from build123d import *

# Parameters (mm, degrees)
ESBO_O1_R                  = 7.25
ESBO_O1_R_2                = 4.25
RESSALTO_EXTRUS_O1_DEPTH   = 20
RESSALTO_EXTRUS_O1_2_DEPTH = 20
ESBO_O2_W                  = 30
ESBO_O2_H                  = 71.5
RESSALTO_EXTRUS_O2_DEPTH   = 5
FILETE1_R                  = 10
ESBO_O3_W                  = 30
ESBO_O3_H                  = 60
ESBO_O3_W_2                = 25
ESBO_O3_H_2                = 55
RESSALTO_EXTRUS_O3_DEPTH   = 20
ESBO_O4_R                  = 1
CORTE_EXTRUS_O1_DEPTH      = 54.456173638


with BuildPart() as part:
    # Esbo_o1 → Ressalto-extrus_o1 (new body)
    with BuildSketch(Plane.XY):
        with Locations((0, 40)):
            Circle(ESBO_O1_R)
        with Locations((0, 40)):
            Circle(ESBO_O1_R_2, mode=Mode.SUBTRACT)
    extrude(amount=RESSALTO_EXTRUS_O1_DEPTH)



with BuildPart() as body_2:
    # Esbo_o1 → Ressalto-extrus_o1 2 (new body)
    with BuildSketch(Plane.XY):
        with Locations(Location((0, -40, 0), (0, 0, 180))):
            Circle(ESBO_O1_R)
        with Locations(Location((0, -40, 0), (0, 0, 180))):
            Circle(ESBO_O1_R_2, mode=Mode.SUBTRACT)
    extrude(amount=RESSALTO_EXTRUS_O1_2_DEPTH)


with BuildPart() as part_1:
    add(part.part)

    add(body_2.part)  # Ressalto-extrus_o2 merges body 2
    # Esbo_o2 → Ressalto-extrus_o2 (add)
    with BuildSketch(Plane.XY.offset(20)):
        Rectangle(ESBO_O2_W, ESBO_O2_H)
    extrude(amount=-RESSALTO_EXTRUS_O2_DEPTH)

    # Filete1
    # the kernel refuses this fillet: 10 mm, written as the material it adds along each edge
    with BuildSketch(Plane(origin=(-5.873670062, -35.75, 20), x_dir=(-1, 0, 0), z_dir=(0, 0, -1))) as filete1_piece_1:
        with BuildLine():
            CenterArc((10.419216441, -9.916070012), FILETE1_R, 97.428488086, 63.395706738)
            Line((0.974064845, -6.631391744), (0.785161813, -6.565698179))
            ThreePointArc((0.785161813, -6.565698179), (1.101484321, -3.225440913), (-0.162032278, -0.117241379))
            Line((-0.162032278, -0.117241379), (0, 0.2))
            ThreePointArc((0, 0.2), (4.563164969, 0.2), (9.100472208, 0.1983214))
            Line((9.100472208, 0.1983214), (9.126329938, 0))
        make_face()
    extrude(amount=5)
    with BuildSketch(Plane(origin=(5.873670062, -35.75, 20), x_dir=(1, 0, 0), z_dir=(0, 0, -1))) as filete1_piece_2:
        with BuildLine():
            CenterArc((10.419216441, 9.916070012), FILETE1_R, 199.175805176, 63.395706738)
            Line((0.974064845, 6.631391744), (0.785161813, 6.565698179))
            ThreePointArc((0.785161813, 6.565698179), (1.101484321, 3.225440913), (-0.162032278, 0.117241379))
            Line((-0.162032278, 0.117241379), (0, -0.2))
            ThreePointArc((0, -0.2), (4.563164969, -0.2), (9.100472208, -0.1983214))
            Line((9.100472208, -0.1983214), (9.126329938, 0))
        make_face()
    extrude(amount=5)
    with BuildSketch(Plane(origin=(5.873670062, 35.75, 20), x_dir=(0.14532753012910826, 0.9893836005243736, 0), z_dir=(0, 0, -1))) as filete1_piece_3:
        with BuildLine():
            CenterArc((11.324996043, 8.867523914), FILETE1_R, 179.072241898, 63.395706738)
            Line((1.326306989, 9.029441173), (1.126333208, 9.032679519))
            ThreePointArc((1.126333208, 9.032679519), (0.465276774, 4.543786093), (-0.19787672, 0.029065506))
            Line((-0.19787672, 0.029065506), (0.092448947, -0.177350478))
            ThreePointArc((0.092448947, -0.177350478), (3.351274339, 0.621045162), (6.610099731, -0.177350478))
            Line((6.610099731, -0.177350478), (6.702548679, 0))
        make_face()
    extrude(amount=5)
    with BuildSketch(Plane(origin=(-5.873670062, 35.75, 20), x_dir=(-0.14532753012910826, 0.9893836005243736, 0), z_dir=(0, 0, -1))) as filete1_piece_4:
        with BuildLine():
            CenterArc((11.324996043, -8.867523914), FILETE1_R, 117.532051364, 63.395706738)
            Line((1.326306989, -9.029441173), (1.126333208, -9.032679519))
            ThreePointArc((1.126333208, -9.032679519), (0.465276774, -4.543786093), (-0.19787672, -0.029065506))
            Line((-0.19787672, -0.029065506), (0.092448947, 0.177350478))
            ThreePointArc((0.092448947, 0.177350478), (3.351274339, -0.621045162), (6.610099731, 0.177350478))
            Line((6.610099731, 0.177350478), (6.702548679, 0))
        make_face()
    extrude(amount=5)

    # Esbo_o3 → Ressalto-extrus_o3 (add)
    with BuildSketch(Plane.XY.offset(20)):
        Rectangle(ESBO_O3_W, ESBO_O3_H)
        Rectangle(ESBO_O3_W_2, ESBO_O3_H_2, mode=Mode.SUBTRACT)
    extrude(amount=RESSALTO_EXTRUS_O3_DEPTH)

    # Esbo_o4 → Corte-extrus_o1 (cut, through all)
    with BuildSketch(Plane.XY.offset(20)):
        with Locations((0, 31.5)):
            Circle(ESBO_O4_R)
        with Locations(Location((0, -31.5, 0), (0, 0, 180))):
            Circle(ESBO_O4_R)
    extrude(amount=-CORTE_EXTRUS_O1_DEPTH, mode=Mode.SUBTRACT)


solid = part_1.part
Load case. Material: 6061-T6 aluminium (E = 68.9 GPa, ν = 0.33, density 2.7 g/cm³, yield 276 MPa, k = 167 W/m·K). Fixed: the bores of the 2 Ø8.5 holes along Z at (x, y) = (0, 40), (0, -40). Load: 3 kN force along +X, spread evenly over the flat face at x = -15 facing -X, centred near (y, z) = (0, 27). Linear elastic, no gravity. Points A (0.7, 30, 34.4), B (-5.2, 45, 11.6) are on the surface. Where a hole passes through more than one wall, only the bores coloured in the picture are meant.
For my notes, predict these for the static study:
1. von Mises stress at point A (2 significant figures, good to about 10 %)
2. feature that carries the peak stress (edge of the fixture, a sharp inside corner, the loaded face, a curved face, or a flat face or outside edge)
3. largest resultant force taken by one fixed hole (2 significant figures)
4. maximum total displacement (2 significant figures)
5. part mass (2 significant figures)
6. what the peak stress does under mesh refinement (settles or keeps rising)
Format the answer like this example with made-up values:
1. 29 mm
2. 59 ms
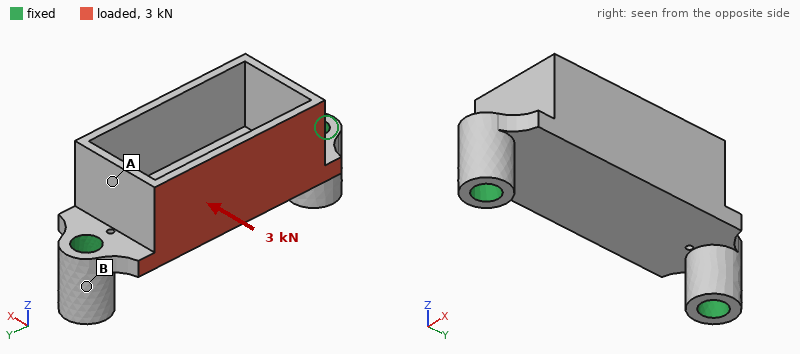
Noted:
1. 30 MPa
2. edge of the fixture
3. 1.5 kN
4. 0.42 mm
5. 64 g
6. keeps rising
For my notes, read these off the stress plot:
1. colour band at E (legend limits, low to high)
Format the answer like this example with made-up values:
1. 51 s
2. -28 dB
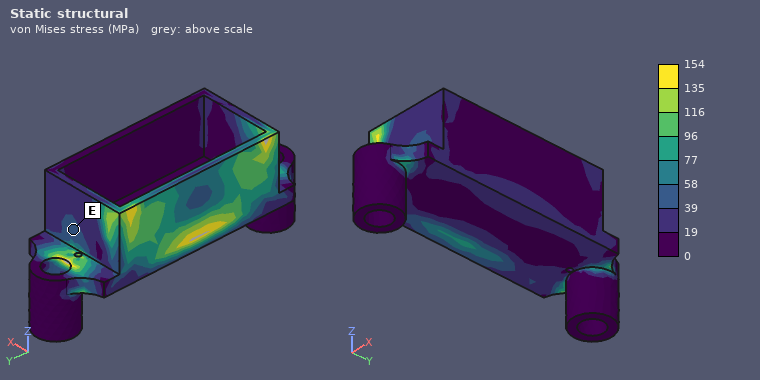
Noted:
1. 39 to 58 MPa
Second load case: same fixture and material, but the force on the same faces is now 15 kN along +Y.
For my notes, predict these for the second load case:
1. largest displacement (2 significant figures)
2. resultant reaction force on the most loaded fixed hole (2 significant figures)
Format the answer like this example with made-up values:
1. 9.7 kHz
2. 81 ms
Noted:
1. 0.15 mm
2. 8.3 kN
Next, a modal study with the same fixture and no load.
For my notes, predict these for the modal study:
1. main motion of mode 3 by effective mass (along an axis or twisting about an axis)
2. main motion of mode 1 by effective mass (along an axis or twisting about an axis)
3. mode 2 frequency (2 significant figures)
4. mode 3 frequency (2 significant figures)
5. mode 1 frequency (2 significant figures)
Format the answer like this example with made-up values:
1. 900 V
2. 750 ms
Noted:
1. along Z
2. along X
3. 6300 Hz
4. 7800 Hz
5. 4400 Hz
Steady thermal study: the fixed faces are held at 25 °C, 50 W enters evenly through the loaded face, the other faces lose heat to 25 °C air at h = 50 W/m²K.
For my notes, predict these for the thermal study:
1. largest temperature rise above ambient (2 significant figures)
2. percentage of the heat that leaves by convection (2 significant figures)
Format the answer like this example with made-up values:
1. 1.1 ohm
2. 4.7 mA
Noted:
1. 34 K
2. 15 %
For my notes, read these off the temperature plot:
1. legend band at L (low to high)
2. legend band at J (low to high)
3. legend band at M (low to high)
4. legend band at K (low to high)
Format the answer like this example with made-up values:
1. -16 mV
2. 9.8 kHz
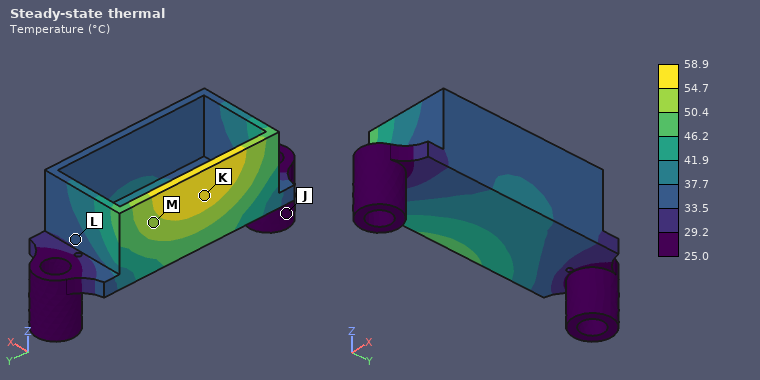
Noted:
1. 33.5 to 37.7 °C
2. 25.0 to 29.2 °C
3. 50.4 to 54.7 °C
4. 54.7 to 58.9 °C
